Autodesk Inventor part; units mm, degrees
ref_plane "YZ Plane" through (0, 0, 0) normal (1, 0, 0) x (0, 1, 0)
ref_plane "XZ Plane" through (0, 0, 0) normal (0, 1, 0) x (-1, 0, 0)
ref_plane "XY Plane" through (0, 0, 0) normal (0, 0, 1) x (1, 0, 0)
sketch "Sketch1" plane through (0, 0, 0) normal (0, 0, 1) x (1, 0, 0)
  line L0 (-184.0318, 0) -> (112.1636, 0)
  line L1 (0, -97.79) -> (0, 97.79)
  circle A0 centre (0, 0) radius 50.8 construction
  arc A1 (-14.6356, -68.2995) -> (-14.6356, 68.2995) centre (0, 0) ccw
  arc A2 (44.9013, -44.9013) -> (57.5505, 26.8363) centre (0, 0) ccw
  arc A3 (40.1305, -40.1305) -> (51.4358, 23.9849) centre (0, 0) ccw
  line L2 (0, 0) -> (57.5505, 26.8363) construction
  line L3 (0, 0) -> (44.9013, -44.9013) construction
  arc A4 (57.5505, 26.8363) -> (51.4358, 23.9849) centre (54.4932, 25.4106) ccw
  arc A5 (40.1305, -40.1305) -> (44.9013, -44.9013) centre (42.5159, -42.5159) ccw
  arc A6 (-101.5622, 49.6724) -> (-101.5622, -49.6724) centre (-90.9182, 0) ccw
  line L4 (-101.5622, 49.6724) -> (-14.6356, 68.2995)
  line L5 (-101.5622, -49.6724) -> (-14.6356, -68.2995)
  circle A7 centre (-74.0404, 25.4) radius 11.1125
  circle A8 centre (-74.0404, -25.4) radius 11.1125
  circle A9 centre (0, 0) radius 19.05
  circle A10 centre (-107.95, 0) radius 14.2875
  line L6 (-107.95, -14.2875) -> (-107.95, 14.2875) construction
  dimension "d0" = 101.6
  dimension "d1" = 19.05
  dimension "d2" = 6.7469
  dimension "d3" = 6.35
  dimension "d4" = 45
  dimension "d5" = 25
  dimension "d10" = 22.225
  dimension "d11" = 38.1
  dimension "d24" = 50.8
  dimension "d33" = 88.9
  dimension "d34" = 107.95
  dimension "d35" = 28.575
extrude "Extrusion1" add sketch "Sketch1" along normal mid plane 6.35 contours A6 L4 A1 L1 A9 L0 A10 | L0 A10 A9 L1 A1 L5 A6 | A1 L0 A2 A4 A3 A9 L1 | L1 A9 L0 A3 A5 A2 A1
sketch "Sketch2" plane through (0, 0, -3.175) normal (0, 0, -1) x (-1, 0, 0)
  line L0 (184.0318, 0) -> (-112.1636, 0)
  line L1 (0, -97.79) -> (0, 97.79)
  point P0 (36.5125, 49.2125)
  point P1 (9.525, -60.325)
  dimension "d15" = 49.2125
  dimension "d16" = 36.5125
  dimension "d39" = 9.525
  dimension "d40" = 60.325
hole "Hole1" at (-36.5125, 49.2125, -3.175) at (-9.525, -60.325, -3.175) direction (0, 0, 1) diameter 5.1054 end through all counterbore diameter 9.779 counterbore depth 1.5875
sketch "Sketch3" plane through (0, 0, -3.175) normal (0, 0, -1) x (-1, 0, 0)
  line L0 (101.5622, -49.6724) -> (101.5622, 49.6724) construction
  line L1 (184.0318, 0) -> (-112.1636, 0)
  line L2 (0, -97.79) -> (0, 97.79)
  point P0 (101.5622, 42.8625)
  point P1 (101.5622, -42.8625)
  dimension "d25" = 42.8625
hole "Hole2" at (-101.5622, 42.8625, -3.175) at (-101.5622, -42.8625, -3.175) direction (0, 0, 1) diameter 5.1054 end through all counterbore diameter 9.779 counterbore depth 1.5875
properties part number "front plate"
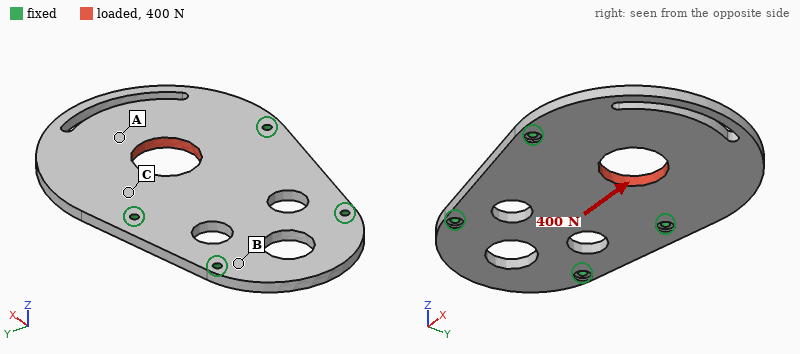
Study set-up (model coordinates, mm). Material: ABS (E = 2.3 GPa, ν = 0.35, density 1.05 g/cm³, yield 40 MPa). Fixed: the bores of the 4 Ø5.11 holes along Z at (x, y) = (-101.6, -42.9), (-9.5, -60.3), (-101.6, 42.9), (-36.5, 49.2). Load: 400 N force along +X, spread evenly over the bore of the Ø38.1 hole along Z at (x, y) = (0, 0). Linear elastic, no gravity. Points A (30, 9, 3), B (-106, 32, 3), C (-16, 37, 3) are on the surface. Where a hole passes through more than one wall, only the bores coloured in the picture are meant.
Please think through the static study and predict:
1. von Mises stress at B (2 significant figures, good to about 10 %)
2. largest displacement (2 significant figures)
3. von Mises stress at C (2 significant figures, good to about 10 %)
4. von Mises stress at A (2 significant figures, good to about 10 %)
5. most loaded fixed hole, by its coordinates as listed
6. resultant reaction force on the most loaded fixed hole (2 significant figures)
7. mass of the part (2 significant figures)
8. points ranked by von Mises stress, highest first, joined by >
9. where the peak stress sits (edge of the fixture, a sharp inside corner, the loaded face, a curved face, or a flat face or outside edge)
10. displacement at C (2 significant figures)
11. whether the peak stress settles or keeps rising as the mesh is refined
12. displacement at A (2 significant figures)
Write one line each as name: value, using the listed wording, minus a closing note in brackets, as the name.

von Mises stress at B: 0.18 MPa
largest displacement: 39 µm
von Mises stress at C: 0.79 MPa
von Mises stress at A: 0.51 MPa
most loaded fixed hole, by its coordinates as listed: (-36.5, 49.2)
resultant reaction force on the most loaded fixed hole: 160 N
mass of the part: 130 g
points ranked by von Mises stress, highest first, joined by >: C > A > B
where the peak stress sits: edge of the fixture
displacement at C: 14 µm
whether the peak stress settles or keeps rising as the mesh is refined: keeps rising
displacement at A: 33 µm
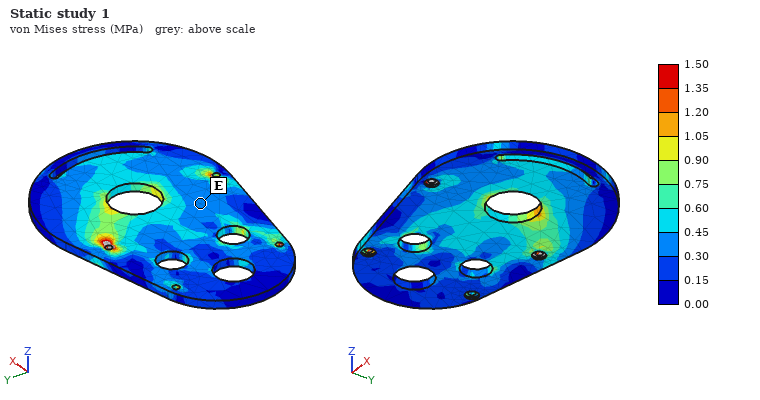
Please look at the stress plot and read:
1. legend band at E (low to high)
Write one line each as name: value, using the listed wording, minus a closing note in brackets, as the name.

legend band at E: 0.30 to 0.45 MPa
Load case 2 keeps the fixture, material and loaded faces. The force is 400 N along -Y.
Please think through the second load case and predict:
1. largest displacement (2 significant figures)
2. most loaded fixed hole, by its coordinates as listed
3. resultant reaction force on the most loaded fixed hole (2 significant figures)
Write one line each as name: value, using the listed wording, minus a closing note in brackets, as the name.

largest displacement: 48 µm
most loaded fixed hole, by its coordinates as listed: (-9.5, -60.3)
resultant reaction force on the most loaded fixed hole: 220 N
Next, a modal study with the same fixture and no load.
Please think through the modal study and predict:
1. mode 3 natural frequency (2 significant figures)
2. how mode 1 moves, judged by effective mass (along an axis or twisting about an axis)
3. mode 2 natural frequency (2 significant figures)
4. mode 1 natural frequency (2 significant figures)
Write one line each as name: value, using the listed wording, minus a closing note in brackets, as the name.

mode 3 natural frequency: 620 Hz
how mode 1 moves, judged by effective mass: along Z
mode 2 natural frequency: 450 Hz
mode 1 natural frequency: 170 Hz
